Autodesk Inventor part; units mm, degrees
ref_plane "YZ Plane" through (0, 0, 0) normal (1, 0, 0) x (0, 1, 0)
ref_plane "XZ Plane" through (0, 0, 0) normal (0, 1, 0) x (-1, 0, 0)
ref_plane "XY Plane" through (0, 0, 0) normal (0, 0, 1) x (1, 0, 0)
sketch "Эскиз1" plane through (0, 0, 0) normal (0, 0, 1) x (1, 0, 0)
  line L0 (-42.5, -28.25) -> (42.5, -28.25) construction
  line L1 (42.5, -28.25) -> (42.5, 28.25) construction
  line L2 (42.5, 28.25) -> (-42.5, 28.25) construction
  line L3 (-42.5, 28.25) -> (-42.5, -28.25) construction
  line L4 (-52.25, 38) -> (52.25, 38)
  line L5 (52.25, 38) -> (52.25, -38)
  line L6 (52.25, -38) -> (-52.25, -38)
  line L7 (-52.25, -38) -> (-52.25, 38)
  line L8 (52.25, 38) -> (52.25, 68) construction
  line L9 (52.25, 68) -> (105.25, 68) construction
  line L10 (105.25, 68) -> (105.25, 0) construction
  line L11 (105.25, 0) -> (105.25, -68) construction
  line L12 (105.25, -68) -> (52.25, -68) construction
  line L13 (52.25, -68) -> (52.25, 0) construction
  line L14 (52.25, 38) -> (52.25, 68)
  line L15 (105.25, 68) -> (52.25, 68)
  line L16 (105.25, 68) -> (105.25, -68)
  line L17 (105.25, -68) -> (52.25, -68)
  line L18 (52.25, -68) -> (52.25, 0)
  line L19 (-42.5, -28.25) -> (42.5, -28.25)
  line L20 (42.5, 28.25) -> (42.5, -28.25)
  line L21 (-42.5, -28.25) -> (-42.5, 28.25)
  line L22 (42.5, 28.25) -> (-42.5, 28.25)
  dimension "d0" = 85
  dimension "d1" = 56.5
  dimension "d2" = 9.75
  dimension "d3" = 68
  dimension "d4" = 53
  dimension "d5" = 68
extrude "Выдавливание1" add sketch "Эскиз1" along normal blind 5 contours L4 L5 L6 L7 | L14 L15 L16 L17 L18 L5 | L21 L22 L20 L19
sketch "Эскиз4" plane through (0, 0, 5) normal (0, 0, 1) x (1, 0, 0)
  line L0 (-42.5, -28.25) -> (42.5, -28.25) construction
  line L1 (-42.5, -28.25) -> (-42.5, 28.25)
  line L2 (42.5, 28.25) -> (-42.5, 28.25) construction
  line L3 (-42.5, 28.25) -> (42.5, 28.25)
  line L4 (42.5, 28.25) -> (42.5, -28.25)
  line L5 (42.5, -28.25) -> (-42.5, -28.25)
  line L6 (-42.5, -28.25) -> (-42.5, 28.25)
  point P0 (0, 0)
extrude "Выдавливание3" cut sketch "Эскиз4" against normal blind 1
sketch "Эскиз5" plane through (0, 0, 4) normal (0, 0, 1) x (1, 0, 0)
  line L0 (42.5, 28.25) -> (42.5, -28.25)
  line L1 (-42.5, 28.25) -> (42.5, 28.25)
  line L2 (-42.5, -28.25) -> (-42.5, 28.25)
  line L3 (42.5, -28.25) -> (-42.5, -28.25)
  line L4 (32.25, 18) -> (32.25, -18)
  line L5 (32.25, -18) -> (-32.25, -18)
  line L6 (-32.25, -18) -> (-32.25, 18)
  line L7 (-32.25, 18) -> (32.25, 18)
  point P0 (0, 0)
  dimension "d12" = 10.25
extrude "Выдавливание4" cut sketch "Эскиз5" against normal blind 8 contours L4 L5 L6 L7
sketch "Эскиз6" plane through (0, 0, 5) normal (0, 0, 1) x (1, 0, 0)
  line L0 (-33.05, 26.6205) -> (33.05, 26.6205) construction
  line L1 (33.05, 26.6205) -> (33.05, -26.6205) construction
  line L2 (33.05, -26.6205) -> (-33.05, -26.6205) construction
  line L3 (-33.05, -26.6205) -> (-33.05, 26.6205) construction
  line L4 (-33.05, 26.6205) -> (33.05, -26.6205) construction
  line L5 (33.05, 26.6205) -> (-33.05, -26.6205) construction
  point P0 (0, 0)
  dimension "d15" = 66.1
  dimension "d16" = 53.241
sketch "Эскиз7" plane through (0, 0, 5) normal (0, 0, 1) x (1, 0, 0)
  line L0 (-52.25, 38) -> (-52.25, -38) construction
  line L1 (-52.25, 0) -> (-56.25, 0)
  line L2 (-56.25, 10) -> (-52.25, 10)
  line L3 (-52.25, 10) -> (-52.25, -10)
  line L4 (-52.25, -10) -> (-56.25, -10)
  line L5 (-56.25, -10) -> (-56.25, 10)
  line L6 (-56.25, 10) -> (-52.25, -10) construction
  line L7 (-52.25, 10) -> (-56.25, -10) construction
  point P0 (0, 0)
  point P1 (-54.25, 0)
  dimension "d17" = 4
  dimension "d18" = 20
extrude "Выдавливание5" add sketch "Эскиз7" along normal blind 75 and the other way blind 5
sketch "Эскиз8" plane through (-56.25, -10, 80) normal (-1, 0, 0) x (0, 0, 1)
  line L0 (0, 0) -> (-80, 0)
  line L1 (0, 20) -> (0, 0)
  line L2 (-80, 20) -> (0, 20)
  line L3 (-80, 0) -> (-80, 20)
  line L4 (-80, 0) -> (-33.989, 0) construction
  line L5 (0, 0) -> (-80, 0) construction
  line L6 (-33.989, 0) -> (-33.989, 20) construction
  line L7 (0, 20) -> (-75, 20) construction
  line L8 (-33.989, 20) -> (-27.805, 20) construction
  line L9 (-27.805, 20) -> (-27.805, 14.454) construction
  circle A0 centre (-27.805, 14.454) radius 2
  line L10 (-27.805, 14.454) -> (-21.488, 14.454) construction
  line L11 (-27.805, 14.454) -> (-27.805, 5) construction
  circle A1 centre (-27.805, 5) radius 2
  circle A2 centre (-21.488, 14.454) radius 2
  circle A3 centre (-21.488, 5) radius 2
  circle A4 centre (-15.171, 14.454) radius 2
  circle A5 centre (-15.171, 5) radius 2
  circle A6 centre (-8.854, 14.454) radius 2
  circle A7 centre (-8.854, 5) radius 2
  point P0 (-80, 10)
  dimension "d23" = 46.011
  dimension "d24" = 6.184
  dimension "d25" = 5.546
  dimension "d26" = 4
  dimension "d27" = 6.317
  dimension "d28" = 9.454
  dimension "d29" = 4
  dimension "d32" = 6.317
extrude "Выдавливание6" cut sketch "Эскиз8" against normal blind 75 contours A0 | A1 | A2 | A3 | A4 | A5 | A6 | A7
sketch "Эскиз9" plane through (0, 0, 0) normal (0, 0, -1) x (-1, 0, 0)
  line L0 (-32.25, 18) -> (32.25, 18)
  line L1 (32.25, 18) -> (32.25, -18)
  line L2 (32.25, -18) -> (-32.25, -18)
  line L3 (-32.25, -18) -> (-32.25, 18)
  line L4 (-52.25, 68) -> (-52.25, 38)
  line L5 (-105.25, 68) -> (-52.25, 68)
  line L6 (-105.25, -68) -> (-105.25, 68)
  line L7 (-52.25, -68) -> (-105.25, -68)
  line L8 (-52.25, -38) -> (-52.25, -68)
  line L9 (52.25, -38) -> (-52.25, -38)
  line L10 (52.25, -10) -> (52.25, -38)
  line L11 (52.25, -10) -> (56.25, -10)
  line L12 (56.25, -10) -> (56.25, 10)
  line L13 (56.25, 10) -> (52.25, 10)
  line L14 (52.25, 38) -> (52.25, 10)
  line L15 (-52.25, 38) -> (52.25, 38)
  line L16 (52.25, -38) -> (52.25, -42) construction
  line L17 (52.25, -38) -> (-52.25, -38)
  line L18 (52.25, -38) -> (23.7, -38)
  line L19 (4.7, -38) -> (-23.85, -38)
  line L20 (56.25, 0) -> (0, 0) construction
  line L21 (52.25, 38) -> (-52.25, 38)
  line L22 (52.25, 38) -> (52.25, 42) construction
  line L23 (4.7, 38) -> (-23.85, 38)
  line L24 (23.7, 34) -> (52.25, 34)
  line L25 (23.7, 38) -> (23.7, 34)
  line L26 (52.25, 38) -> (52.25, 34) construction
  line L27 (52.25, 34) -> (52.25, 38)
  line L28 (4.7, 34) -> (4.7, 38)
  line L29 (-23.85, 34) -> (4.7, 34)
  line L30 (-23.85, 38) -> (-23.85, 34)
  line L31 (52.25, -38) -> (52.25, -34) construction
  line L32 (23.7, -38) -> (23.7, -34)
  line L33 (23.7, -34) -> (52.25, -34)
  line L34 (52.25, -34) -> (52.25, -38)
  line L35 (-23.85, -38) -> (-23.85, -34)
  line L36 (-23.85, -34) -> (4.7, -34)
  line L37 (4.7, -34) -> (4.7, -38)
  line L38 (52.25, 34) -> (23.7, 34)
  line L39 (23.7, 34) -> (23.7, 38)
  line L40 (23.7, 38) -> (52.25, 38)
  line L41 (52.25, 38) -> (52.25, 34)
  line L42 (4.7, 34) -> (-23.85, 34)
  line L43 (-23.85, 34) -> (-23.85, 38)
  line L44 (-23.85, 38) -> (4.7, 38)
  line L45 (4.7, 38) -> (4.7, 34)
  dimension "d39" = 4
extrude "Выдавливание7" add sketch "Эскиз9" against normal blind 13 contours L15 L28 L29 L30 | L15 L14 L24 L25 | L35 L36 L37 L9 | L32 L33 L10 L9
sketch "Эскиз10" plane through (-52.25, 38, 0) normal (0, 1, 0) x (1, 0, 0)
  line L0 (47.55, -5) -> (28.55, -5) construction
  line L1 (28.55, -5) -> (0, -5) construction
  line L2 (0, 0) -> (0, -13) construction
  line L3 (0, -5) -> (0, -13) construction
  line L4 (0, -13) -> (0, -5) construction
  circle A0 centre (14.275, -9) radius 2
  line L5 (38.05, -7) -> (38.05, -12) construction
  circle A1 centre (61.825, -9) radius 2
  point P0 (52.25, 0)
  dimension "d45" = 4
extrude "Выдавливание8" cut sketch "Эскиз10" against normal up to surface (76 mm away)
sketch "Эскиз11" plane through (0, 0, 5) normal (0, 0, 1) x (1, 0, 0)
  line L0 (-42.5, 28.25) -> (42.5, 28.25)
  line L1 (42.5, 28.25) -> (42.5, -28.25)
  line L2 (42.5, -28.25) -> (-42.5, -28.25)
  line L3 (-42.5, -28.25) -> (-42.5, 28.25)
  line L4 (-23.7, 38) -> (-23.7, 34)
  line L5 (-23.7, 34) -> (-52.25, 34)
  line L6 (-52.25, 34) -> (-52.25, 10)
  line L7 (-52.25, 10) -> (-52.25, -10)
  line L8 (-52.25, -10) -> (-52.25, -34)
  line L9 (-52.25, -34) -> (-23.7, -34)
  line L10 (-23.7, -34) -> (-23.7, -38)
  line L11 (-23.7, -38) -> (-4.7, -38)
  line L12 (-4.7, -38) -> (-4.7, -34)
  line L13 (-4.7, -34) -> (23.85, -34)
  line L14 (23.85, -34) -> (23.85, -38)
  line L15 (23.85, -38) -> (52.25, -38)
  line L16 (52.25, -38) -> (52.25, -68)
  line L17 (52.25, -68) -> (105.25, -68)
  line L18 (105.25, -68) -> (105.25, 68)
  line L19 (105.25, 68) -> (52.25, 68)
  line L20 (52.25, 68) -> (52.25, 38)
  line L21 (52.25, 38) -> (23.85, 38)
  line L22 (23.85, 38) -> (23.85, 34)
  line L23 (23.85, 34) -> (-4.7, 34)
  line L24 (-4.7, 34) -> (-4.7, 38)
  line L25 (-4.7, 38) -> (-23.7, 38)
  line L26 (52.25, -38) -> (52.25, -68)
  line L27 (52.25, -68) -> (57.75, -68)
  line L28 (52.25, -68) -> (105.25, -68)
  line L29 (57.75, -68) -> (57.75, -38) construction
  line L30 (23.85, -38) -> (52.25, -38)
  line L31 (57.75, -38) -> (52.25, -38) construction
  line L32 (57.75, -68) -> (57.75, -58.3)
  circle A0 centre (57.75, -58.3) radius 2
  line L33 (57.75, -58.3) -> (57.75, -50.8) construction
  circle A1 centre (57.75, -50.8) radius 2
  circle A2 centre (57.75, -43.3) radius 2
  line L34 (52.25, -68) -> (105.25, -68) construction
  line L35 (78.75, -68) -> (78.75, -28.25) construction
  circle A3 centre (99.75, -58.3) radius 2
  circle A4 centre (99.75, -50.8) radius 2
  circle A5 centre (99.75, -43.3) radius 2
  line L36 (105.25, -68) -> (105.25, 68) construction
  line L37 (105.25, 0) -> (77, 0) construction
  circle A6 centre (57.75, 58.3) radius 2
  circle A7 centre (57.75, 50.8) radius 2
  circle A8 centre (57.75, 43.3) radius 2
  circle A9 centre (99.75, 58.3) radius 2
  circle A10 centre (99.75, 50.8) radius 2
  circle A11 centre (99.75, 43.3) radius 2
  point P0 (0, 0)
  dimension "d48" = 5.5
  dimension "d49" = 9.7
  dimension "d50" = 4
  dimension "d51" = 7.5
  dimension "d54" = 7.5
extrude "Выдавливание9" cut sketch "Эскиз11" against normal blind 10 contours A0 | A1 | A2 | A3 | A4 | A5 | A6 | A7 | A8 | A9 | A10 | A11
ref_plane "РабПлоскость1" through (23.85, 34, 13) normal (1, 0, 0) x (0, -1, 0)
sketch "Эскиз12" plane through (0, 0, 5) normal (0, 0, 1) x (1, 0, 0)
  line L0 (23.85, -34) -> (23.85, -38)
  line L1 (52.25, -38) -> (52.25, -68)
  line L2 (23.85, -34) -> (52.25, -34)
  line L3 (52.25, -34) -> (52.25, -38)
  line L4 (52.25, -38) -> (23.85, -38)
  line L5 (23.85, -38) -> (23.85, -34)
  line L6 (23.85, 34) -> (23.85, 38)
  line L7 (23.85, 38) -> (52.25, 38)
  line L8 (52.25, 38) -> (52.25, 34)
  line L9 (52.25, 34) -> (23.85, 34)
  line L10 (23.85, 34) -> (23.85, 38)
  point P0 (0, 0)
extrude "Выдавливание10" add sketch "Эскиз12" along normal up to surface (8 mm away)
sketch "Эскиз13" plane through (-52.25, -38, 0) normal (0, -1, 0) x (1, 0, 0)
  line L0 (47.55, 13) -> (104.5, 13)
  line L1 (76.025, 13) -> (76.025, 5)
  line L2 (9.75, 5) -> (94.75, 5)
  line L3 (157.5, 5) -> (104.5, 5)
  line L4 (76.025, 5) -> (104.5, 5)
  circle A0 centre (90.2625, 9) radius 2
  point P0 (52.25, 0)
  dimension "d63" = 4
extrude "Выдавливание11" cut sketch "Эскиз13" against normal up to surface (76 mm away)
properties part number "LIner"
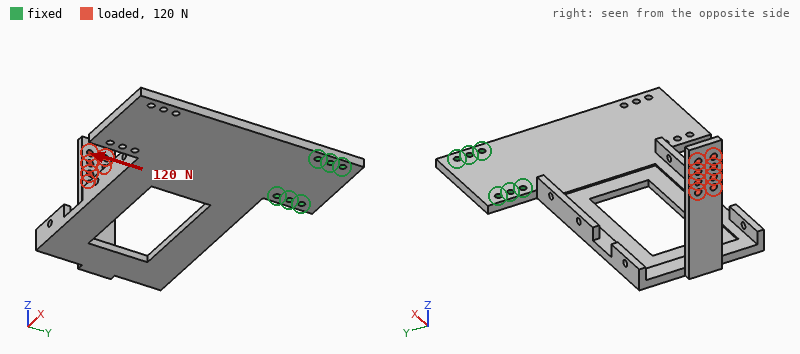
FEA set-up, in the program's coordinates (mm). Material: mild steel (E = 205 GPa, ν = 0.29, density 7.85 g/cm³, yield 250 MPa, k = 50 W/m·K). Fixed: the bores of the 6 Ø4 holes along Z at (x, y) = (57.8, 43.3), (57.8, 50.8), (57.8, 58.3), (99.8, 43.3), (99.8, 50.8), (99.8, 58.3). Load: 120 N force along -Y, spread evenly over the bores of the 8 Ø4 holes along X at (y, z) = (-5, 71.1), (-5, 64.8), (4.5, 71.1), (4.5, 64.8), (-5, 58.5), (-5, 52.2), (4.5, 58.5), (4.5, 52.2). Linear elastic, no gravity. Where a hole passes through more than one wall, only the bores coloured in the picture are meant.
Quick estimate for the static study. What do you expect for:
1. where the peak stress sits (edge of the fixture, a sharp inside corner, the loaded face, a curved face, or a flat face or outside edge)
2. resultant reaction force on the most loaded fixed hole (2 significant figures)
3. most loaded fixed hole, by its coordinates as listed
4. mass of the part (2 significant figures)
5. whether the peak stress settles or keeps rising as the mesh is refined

edge of the fixture
410 N
(57.8, 43.3)
570 g
keeps rising
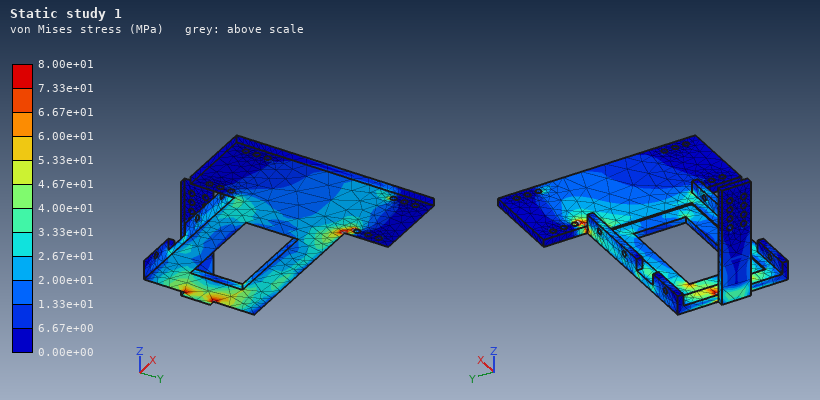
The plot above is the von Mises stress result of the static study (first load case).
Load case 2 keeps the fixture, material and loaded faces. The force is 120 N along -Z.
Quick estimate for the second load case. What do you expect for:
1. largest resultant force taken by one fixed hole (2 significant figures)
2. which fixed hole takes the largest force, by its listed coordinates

550 N
(57.8, 43.3)
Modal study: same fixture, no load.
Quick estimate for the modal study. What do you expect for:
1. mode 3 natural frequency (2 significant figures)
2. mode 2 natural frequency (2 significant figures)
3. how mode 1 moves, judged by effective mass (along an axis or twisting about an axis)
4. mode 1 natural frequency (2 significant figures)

490 Hz
290 Hz
along Z
200 Hz
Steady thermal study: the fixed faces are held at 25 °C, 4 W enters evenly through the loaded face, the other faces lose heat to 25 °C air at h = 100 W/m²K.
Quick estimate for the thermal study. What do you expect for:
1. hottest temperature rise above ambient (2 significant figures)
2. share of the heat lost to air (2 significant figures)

18 K
100 %
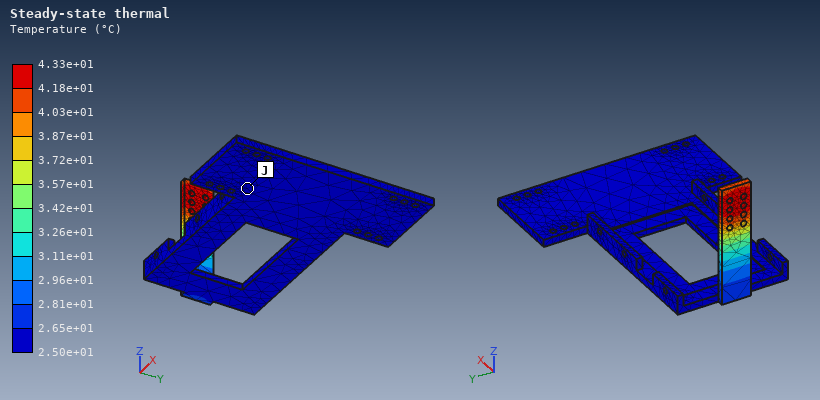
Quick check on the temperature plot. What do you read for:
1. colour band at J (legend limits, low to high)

2.50e+01 to 2.65e+01 °C
